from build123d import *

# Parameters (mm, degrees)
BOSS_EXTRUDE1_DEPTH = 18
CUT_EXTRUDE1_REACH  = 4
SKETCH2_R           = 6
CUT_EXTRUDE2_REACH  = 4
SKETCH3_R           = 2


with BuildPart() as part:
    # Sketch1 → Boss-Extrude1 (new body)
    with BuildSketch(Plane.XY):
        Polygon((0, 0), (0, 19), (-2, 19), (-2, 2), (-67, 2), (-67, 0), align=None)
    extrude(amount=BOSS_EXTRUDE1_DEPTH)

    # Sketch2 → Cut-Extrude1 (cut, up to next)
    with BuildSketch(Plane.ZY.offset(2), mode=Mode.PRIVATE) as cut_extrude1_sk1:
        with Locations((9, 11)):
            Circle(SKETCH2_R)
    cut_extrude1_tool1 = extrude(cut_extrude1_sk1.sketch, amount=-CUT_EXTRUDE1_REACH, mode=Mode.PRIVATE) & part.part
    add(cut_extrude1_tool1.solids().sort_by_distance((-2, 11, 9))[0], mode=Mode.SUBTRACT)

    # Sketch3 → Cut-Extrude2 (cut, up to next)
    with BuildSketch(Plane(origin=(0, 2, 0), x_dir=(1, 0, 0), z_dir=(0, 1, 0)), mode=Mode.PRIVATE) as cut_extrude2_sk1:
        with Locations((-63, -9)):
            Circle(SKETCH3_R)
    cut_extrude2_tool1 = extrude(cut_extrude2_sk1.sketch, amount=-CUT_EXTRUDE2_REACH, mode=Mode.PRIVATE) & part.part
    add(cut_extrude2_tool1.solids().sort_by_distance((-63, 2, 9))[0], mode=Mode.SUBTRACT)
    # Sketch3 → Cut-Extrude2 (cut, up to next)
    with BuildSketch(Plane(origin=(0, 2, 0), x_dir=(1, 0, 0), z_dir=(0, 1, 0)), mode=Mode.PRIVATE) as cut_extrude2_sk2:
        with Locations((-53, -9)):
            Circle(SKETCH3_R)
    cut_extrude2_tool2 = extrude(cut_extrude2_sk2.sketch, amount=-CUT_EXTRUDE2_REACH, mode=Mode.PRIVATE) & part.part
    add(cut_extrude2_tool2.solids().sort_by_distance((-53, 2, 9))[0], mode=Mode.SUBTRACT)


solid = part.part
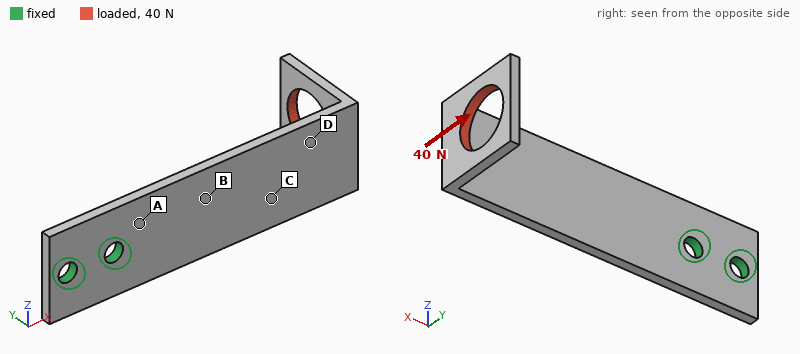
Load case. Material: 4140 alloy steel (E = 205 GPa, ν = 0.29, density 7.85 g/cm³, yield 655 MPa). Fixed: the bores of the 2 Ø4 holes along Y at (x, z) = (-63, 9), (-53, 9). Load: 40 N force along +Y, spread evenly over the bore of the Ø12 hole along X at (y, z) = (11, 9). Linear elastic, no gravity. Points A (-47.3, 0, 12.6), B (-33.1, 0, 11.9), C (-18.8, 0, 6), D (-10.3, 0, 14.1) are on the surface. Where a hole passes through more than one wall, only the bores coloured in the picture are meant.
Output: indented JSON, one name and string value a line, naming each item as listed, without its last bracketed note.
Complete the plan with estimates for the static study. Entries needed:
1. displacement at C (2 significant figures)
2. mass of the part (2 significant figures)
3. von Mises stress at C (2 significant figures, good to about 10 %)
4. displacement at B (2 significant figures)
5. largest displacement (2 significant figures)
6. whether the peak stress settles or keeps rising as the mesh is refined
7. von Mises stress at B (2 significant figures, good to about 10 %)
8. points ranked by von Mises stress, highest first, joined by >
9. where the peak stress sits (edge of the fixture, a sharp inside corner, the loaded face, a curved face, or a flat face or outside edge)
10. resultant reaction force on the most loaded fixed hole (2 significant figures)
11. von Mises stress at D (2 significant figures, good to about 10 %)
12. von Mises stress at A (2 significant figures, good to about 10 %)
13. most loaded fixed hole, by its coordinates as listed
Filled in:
{
  "displacement at C": "0.36 mm",
  "mass of the part": "22 g",
  "von Mises stress at C": "59 MPa",
  "displacement at B": "0.13 mm",
  "largest displacement": "0.83 mm",
  "whether the peak stress settles or keeps rising as the mesh is refined": "keeps rising",
  "von Mises stress at B": "100 MPa",
  "points ranked by von Mises stress, highest first, joined by >": "A > B > C > D",
  "where the peak stress sits": "edge of the fixture",
  "resultant reaction force on the most loaded fixed hole": "84 N",
  "von Mises stress at D": "32 MPa",
  "von Mises stress at A": "150 MPa",
  "most loaded fixed hole, by its coordinates as listed": "(-53, 9)"
}
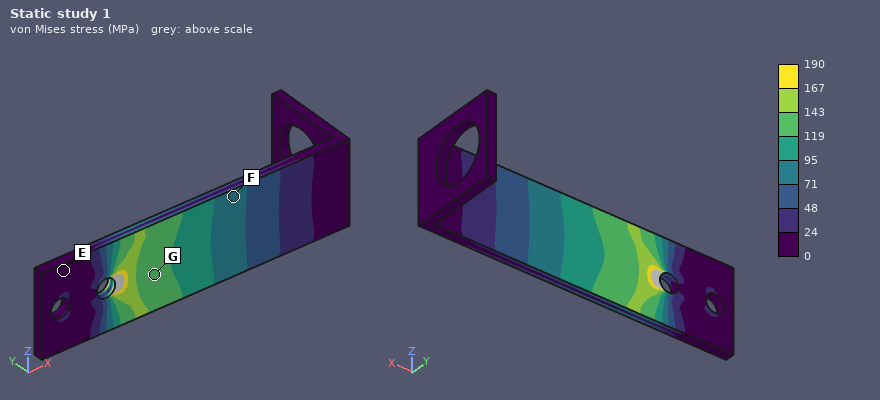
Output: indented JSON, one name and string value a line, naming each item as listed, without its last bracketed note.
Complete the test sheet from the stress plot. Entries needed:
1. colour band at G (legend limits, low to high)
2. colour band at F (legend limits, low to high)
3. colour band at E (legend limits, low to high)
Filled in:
{
  "colour band at G": "119 to 143 MPa",
  "colour band at F": "71 to 95 MPa",
  "colour band at E": "0 to 24 MPa"
}
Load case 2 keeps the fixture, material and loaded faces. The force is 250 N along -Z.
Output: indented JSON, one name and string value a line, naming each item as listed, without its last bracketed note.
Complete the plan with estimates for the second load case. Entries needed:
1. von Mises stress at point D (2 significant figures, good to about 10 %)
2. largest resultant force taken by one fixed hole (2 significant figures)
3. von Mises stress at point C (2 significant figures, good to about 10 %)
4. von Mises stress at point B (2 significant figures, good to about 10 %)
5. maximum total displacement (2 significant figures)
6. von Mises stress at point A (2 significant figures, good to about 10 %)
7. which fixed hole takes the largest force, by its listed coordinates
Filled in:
{
  "von Mises stress at point D": "170 MPa",
  "largest resultant force taken by one fixed hole": "1.0 kN",
  "von Mises stress at point C": "180 MPa",
  "von Mises stress at point B": "180 MPa",
  "maximum total displacement": "0.77 mm",
  "von Mises stress at point A": "150 MPa",
  "which fixed hole takes the largest force, by its listed coordinates": "(-53, 9)"
}
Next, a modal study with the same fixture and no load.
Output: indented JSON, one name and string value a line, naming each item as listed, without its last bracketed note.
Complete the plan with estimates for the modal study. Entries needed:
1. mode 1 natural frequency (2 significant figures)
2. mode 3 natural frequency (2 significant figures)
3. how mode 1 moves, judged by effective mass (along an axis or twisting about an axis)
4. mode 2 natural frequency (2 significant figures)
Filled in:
{
  "mode 1 natural frequency": "450 Hz",
  "mode 3 natural frequency": "2300 Hz",
  "how mode 1 moves, judged by effective mass": "along Y",
  "mode 2 natural frequency": "1700 Hz"
}
